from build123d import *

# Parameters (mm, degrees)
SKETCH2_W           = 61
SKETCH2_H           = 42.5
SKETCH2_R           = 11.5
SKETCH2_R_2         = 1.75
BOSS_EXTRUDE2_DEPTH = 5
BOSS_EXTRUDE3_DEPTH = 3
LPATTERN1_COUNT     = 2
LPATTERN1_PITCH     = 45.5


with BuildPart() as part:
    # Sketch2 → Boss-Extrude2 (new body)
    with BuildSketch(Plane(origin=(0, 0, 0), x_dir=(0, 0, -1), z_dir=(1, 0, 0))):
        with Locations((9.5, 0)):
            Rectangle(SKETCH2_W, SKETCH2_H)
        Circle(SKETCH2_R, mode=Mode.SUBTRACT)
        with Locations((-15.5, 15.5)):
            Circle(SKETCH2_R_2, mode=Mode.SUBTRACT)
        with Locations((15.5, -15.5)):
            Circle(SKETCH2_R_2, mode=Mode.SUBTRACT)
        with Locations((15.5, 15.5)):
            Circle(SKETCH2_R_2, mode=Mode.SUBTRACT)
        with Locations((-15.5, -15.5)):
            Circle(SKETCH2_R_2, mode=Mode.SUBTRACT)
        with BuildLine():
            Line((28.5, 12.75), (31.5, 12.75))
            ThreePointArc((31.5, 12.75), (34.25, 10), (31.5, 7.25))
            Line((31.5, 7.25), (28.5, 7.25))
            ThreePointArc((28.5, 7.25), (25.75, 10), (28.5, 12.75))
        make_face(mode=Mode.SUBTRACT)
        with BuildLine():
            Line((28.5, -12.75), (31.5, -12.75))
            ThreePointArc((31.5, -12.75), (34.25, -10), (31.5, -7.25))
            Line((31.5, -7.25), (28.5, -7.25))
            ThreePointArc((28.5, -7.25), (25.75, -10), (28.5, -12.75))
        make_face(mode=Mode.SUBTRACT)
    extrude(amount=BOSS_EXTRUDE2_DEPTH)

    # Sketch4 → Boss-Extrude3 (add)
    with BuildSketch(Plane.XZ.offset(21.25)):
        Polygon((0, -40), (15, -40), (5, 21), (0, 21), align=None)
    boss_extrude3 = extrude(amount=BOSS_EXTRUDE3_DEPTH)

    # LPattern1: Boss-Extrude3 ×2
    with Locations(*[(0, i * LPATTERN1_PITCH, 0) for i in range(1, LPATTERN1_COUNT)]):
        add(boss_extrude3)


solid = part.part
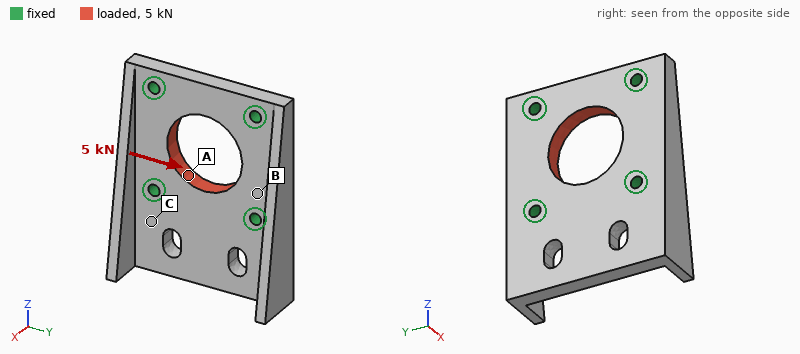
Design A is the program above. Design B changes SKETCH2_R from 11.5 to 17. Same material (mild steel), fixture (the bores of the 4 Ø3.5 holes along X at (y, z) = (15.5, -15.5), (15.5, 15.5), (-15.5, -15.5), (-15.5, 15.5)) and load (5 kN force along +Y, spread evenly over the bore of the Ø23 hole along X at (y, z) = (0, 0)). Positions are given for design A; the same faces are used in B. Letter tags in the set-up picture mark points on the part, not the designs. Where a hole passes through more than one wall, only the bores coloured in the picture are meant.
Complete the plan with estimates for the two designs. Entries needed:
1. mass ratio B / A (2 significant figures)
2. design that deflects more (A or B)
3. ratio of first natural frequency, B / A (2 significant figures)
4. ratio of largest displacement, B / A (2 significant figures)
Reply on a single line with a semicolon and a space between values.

0.82; B; 0.96; 1.3
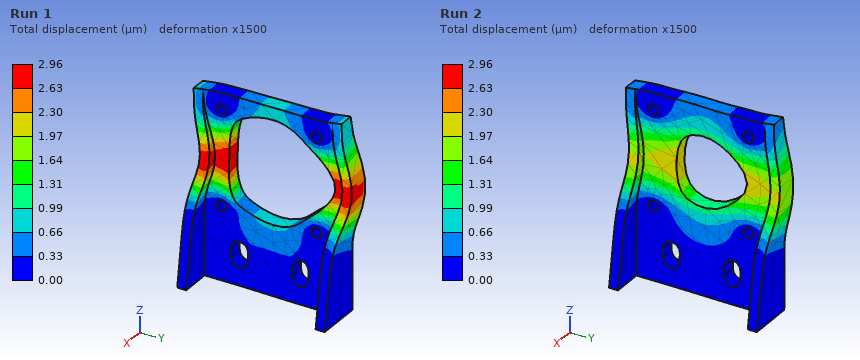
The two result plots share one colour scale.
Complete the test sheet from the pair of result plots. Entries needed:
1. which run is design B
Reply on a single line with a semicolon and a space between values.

Run 1
